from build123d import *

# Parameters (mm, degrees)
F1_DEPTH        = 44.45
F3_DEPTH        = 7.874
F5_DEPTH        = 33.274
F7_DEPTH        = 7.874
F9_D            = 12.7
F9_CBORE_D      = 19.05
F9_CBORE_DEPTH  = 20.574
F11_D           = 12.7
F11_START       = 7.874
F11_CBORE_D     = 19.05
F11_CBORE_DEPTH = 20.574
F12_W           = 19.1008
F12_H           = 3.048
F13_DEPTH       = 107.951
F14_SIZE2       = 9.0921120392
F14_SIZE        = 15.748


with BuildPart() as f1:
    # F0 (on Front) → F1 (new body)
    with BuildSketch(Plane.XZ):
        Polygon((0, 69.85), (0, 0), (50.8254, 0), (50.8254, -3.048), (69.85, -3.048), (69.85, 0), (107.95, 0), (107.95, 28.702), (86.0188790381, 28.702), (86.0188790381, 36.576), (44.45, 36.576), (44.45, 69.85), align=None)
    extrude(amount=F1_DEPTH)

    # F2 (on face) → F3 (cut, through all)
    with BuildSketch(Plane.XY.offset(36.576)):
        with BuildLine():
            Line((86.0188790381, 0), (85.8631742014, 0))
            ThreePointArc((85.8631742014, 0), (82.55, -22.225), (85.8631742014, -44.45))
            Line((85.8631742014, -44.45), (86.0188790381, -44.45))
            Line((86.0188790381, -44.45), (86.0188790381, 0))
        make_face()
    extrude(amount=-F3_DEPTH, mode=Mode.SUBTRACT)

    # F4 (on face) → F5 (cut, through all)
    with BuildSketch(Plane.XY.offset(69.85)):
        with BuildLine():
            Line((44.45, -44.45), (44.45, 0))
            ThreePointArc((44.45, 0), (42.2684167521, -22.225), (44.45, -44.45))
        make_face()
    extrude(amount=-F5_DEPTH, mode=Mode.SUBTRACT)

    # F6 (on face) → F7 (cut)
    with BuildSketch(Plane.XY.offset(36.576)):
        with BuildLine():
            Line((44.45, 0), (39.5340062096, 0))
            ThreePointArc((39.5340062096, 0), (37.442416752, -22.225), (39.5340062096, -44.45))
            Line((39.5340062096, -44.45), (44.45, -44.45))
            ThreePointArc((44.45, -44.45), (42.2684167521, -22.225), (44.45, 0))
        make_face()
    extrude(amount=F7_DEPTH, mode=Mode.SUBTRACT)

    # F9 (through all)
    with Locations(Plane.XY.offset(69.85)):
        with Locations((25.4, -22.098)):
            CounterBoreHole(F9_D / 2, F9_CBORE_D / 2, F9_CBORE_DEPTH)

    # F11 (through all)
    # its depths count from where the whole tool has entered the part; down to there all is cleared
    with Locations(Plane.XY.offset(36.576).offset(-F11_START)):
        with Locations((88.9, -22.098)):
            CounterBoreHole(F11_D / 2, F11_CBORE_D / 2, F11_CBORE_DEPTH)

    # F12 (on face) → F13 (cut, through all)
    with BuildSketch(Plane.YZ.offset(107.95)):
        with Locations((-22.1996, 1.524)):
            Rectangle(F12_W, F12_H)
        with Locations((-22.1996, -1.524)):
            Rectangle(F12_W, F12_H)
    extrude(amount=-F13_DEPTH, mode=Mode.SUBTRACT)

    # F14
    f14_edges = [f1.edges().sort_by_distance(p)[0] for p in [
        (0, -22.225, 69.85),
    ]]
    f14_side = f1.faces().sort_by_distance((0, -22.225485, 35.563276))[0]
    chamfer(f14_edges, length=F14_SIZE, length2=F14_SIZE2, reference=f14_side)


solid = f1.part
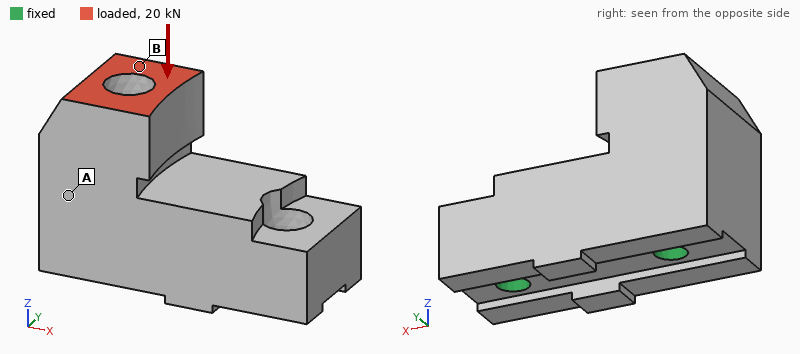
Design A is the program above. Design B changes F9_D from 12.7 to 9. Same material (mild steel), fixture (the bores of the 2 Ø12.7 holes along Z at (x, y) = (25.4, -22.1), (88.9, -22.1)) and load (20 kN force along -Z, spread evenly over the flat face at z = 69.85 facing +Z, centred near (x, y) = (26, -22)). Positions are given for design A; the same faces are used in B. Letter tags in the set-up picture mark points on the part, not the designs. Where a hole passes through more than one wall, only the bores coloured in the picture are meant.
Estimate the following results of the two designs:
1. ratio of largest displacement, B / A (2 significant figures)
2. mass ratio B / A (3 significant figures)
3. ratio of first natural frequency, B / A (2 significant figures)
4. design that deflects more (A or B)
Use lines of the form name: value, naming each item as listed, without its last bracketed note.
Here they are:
ratio of largest displacement, B / A: 1.1
mass ratio B / A: 1.01
ratio of first natural frequency, B / A: 0.94
design that deflects more: B
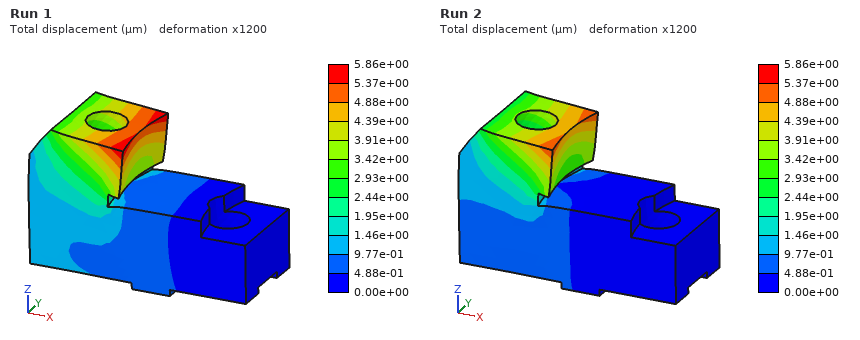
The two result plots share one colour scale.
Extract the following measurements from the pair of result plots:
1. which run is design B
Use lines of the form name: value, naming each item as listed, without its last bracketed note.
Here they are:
which run is design B: Run 1
